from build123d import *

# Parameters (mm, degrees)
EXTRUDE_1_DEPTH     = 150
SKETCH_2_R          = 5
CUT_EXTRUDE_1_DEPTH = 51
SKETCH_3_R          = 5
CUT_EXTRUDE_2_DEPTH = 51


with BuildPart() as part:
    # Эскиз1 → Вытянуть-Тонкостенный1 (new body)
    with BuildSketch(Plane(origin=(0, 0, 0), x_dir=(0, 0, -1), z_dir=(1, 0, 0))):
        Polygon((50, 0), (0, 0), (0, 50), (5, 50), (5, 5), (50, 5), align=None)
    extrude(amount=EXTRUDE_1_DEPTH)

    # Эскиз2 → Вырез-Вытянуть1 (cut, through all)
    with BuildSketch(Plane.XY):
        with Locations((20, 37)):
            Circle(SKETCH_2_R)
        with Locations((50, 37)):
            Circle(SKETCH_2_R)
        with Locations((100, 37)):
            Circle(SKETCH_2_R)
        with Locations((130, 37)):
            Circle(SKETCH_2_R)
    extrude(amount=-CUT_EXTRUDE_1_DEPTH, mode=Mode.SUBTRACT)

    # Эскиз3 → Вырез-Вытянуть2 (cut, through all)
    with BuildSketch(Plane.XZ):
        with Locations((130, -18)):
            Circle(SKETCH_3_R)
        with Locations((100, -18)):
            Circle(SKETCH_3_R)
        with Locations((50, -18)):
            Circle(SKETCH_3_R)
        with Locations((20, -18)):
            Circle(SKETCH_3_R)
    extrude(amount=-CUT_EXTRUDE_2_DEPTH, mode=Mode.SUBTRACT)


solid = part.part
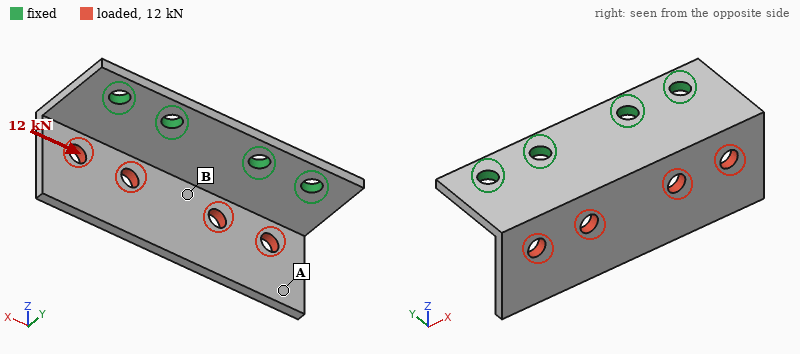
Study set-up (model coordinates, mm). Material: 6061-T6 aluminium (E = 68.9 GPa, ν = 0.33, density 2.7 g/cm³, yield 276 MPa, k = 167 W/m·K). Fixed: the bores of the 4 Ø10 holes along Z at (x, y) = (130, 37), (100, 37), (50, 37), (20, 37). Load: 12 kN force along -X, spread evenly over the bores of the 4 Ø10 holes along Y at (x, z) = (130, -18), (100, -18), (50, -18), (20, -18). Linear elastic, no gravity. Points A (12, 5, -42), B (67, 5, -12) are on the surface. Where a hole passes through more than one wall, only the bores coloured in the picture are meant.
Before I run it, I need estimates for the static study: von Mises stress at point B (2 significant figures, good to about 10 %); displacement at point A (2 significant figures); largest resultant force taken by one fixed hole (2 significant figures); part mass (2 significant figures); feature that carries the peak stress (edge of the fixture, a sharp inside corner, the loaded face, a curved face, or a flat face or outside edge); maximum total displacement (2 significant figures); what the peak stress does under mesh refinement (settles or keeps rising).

73 MPa
0.59 mm
4.2 kN
180 g
edge of the fixture
0.74 mm
keeps rising
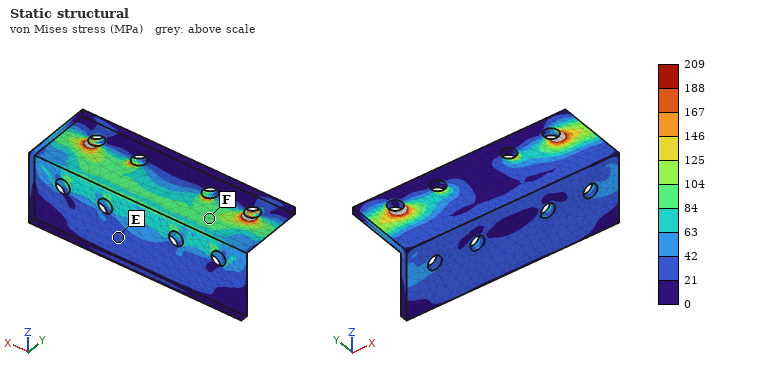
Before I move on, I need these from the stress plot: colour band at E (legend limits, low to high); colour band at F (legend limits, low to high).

21 to 42 MPa
84 to 104 MPa
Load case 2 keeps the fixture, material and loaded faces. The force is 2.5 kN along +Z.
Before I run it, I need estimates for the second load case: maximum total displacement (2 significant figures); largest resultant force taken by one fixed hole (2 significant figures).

0.62 mm
650 N
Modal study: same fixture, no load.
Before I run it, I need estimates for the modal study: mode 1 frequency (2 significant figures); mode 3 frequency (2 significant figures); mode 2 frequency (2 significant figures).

870 Hz
2400 Hz
1300 Hz
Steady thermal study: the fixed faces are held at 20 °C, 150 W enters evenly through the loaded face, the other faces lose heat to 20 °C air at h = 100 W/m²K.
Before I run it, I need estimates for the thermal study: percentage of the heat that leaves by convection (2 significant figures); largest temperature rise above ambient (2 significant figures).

42 %
43 K
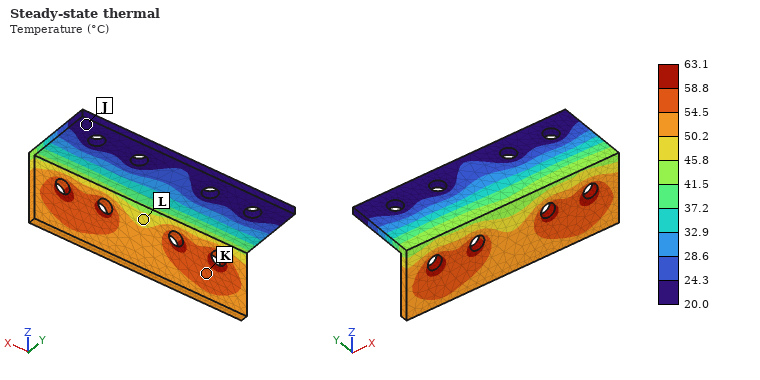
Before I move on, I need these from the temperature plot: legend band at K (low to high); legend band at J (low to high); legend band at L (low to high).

54.5 to 58.8 °C
20.0 to 24.3 °C
45.8 to 50.2 °C
